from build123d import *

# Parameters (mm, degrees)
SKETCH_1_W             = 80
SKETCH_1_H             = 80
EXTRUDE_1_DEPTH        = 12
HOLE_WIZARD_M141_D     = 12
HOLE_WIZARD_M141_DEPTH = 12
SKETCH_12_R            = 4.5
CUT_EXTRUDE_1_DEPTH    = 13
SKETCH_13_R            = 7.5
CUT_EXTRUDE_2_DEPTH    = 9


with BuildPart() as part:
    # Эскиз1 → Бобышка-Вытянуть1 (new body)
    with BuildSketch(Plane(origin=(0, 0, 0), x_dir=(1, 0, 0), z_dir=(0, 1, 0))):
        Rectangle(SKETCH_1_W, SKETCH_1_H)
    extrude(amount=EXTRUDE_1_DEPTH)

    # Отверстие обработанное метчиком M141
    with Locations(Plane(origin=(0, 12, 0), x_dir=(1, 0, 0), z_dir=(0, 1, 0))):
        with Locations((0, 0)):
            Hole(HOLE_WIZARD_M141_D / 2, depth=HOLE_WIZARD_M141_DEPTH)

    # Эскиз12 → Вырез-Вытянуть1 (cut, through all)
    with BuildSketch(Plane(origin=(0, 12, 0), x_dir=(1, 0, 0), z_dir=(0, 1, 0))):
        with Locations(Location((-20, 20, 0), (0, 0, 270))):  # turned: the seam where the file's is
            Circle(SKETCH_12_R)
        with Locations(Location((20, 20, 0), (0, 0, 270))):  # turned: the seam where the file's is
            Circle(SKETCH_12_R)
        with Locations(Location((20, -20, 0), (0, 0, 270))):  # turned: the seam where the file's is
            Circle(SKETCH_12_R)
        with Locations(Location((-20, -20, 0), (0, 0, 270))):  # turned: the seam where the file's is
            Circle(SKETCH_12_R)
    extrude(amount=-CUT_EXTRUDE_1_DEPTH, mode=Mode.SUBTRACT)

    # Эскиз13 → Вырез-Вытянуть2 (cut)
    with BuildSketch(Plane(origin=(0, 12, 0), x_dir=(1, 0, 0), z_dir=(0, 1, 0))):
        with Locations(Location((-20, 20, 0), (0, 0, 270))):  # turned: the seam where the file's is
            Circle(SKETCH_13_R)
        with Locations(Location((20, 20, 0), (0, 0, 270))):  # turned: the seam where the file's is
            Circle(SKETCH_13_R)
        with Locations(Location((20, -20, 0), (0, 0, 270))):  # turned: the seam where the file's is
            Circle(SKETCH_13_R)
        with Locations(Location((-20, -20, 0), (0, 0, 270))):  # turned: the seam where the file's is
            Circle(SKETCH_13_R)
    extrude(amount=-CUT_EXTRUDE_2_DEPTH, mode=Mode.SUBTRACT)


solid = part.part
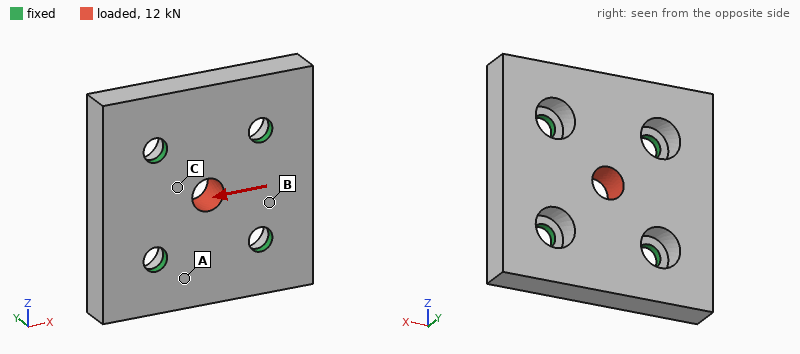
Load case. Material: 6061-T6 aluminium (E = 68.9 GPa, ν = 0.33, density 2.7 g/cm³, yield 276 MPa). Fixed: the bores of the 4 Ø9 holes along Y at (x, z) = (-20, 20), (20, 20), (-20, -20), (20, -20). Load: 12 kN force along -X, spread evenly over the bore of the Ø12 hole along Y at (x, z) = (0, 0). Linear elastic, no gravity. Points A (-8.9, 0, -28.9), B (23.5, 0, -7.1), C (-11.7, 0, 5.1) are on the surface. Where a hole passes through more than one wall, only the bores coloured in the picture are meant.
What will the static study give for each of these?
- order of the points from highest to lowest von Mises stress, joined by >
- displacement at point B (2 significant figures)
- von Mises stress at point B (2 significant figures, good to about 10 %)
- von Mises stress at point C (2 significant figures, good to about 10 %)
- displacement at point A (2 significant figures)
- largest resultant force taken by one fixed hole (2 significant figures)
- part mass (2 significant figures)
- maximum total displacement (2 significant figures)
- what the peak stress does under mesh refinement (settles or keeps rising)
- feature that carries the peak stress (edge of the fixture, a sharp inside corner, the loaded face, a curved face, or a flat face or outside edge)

C > B > A
5.9 µm
13 MPa
21 MPa
2.4 µm
3.1 kN
180 g
13 µm
keeps rising
edge of the fixture
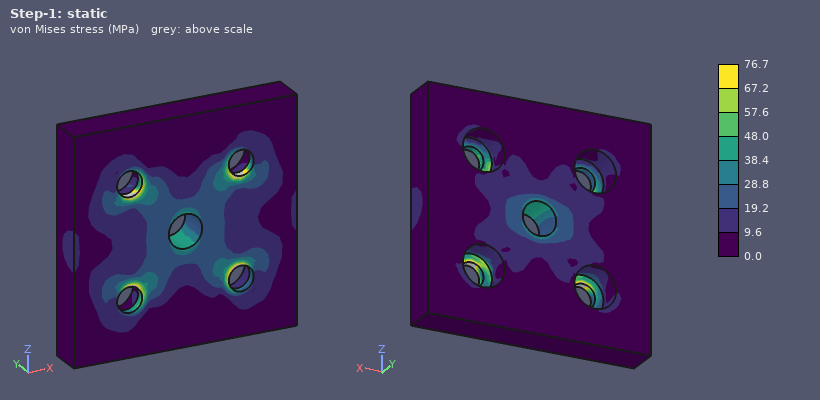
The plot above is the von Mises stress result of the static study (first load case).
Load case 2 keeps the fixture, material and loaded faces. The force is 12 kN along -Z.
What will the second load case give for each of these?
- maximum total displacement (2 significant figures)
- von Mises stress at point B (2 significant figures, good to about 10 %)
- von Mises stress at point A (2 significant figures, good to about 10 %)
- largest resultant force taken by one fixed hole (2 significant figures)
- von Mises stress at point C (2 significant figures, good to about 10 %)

13 µm
9.6 MPa
14 MPa
3.1 kN
20 MPa
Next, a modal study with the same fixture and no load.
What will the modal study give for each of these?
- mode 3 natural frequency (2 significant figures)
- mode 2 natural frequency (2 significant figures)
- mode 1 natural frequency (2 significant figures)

11 kHz
9800 Hz
9800 Hz
